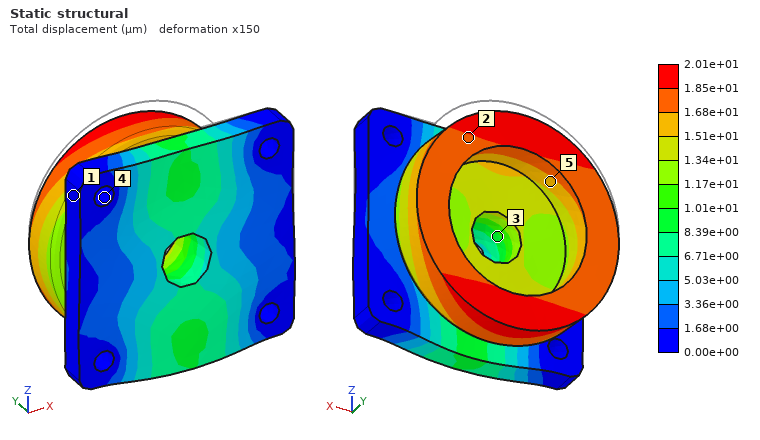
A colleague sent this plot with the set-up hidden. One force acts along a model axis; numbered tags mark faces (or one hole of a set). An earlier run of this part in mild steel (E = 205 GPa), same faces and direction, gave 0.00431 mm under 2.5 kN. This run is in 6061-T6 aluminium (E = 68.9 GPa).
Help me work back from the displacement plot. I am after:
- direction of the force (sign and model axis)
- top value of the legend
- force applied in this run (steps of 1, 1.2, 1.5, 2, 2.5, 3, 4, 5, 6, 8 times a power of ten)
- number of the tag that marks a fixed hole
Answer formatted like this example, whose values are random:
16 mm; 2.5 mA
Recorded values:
-Z; 2.01e+01 µm; 4 kN; 4
